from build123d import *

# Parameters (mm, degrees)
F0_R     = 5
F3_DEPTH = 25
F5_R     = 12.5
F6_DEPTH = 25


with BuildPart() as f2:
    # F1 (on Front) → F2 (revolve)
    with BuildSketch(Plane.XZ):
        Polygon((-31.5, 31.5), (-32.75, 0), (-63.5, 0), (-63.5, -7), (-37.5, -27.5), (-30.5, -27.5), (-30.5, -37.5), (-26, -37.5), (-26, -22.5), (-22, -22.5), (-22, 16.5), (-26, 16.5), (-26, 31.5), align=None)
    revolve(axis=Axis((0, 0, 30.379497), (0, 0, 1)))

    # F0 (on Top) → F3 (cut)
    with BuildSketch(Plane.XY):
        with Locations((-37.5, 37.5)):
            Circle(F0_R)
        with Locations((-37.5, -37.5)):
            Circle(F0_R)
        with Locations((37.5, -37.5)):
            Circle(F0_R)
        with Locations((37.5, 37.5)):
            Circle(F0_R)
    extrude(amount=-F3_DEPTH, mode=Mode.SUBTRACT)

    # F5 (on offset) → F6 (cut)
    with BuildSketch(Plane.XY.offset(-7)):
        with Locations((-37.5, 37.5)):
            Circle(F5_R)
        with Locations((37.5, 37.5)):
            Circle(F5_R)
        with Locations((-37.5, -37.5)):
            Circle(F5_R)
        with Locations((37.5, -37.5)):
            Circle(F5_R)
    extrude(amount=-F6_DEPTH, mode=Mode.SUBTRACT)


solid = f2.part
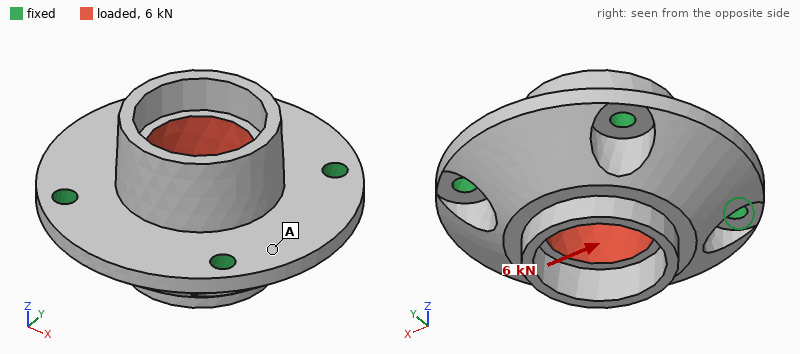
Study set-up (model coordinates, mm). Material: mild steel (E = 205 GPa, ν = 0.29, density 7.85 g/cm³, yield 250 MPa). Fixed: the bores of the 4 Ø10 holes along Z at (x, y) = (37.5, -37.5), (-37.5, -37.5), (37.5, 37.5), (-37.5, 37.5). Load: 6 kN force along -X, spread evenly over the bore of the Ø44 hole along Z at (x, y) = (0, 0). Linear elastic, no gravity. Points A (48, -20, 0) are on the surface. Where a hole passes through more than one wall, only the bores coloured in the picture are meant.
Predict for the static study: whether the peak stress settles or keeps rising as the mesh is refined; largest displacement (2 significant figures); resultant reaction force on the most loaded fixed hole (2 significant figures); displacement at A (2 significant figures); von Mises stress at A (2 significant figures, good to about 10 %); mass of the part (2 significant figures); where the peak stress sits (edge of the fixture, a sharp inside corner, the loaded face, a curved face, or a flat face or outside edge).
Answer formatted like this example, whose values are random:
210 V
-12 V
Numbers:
keeps rising
1.5 µm
1.5 kN
0.63 µm
2.4 MPa
1.9 kg
edge of the fixture
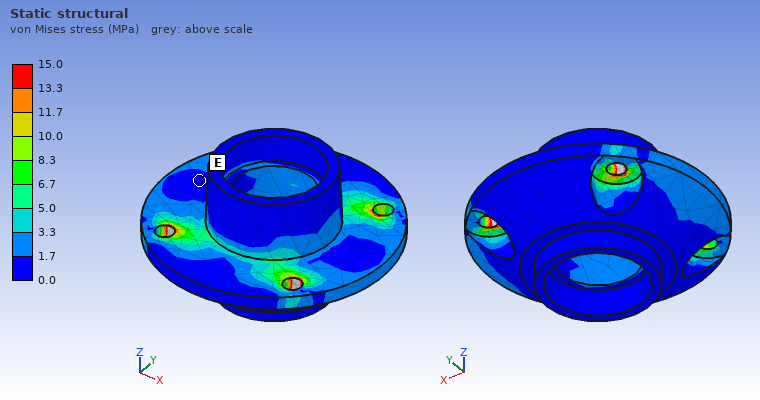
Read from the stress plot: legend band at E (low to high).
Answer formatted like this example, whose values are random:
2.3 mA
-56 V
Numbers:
0.0 to 1.7 MPa
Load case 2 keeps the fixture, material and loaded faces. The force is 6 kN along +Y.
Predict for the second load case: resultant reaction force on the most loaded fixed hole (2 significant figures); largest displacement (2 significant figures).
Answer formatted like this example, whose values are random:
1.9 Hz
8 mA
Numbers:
1.5 kN
1.5 µm
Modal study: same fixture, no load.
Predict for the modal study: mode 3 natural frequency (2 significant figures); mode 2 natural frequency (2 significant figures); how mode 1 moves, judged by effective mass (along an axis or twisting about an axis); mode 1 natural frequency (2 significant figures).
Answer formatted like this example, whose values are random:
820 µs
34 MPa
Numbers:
7400 Hz
7400 Hz
along Z
6600 Hz
